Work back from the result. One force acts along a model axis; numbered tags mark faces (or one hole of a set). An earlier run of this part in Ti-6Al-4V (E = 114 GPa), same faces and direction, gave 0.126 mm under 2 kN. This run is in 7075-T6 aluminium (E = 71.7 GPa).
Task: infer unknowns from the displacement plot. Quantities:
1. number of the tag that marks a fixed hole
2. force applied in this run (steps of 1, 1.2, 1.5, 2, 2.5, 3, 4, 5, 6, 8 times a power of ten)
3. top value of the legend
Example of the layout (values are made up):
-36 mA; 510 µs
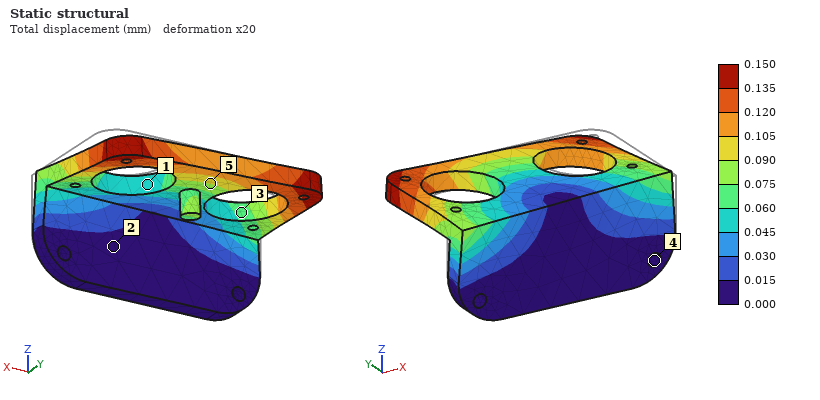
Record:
4; 1.5 kN; 0.150 mm
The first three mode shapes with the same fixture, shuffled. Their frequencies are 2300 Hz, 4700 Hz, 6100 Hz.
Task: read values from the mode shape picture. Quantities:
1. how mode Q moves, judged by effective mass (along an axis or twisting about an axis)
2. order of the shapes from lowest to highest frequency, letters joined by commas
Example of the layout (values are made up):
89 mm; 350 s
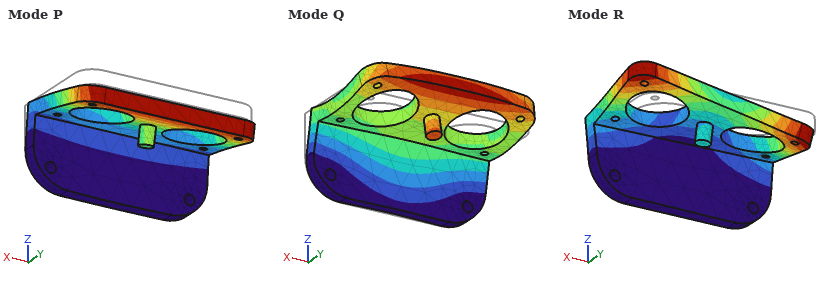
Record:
along Y; P, R, Q
